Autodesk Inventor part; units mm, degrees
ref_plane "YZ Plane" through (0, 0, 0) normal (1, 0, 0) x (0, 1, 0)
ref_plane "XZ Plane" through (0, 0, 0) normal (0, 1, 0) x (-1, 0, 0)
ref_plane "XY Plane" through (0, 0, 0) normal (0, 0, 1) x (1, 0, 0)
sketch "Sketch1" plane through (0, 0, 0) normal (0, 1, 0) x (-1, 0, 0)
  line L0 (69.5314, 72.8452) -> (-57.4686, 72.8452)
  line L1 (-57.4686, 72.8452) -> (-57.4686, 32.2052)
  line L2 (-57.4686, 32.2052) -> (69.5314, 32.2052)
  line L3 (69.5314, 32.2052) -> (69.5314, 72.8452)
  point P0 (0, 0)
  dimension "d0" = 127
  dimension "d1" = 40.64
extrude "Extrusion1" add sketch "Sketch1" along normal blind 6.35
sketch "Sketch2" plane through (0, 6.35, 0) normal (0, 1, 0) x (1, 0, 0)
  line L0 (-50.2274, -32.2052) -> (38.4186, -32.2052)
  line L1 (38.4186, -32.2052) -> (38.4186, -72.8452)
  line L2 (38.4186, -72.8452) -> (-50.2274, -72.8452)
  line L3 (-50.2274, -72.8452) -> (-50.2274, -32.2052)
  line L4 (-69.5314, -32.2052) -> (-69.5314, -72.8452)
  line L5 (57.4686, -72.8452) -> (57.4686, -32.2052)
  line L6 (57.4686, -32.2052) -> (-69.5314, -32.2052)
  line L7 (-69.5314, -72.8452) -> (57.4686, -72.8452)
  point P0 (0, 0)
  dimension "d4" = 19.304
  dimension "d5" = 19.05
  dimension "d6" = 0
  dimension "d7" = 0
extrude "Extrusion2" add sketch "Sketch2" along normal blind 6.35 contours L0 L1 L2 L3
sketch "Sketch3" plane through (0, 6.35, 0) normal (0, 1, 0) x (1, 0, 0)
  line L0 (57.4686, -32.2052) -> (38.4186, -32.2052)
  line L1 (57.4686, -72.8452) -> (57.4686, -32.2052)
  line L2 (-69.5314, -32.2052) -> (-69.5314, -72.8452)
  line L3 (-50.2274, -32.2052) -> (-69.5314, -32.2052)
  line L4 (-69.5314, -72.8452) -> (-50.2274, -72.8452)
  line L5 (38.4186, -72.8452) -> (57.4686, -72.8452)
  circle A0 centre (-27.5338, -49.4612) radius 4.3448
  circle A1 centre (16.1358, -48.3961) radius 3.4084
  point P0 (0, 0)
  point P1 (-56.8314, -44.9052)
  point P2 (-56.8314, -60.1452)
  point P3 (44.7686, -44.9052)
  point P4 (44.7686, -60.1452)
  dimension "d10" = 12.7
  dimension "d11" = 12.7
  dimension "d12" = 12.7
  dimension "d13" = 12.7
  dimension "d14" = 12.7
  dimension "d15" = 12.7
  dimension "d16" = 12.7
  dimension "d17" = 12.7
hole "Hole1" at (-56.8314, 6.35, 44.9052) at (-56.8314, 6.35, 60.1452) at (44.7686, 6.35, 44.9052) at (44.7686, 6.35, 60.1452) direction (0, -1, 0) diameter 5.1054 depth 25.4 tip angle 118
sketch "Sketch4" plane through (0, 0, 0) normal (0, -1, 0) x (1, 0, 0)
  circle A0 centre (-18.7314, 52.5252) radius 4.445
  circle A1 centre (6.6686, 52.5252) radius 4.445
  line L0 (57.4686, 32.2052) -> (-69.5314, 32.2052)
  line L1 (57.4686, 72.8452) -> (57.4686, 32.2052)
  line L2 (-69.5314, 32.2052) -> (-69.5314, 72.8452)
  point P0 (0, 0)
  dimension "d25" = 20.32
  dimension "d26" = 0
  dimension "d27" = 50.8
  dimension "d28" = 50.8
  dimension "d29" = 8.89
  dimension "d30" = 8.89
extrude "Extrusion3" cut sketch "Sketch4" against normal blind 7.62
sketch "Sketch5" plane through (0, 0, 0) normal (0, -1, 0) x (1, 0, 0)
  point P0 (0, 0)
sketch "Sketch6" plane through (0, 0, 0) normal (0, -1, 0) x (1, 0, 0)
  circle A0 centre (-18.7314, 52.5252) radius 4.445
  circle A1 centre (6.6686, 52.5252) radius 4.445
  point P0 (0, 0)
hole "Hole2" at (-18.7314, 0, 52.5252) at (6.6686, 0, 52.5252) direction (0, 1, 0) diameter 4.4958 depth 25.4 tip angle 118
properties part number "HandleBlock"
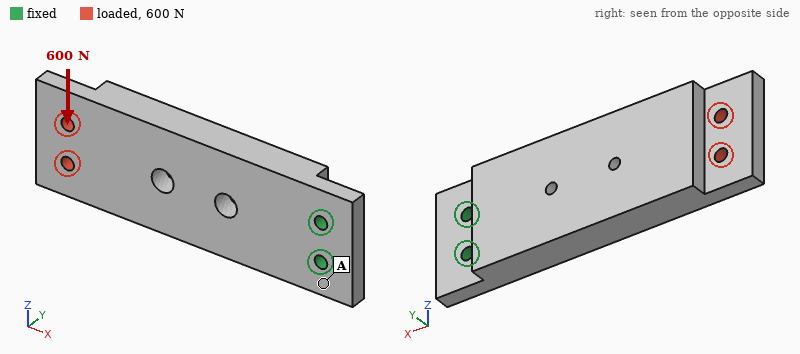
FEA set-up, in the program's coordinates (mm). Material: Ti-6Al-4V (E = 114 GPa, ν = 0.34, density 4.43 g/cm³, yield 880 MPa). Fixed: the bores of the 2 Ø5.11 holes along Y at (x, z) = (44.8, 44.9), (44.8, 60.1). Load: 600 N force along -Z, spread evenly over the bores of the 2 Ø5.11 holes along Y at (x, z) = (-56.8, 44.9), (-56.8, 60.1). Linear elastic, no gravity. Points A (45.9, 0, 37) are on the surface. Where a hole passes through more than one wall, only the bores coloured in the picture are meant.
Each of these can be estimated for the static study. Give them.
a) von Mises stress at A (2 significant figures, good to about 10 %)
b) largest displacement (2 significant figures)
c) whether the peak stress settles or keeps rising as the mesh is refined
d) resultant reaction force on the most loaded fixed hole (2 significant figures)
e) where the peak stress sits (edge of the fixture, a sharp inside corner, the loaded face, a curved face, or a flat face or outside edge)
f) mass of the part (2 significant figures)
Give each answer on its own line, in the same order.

10 MPa
73 µm
keeps rising
3.2 kN
edge of the fixture
240 g
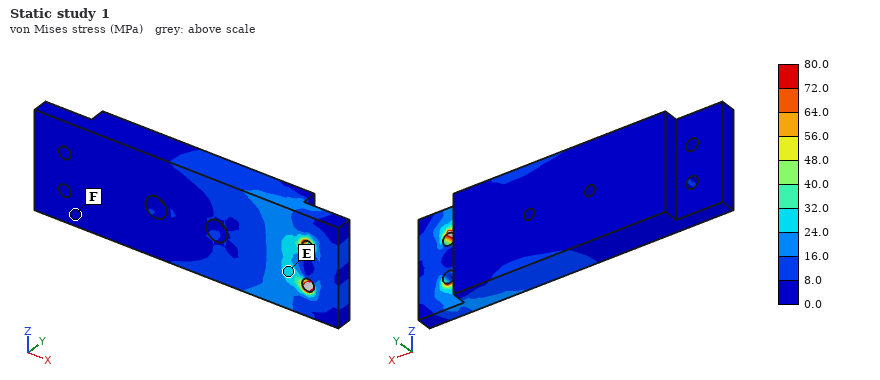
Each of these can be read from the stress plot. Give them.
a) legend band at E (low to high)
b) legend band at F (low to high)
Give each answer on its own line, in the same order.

24.0 to 32.0 MPa
0.0 to 8.0 MPa
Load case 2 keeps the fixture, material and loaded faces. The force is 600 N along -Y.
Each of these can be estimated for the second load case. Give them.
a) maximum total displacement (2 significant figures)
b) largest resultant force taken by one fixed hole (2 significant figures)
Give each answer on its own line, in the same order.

0.82 mm
320 N
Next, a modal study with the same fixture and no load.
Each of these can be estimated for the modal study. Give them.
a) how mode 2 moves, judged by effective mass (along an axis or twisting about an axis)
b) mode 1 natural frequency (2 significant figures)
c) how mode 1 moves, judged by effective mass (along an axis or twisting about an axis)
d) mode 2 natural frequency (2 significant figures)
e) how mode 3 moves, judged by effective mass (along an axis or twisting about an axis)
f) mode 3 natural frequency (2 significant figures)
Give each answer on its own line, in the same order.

along Z
540 Hz
along Y
1800 Hz
twisting about X
3500 Hz
